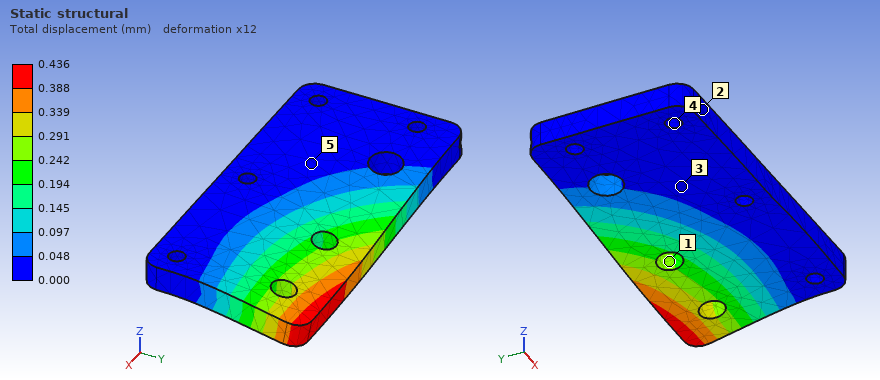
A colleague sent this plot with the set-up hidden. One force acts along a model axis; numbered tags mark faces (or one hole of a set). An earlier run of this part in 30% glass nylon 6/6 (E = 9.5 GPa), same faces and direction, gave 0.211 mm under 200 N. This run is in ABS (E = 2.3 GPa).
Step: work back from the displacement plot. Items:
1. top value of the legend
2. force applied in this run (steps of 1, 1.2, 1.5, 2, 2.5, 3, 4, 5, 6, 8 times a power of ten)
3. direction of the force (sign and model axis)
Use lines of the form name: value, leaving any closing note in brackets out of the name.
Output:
top value of the legend: 0.436 mm
force applied in this run: 100 N
direction of the force: -Z
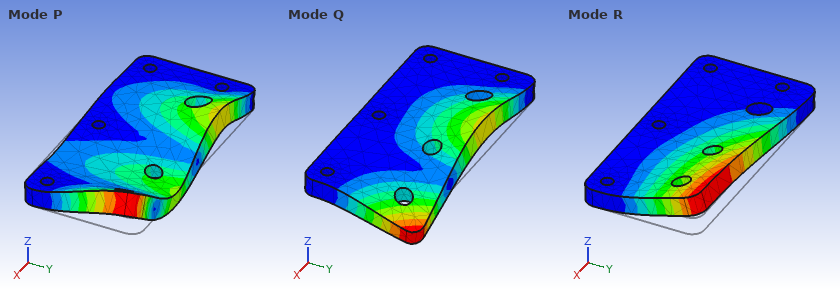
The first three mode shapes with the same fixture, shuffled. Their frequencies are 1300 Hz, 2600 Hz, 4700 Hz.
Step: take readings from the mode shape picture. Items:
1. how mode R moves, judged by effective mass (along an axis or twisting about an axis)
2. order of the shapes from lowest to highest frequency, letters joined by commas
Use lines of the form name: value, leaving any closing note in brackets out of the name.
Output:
how mode R moves, judged by effective mass: along Z
order of the shapes from lowest to highest frequency, letters joined by commas: R, Q, P
